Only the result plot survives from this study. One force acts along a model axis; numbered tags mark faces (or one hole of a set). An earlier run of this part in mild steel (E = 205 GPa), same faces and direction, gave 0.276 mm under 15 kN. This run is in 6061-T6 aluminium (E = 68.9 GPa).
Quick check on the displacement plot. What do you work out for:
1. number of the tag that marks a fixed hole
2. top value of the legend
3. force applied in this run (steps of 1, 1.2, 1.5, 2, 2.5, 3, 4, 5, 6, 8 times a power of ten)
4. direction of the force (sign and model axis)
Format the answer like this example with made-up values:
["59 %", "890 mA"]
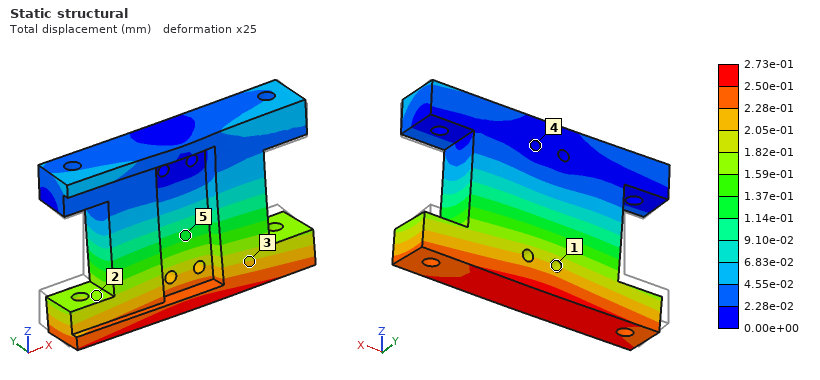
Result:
["4", "2.73e-01 mm", "5 kN", "-Y"]
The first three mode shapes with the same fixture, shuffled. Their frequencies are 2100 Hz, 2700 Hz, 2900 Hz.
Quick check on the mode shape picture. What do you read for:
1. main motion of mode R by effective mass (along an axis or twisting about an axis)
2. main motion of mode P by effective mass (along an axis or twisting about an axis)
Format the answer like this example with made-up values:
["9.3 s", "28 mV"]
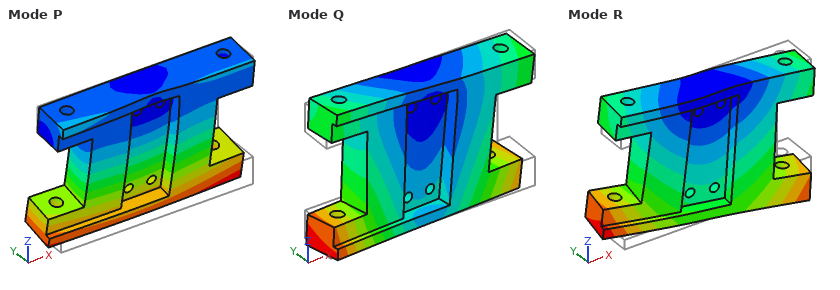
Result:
["along X", "along Y"]
